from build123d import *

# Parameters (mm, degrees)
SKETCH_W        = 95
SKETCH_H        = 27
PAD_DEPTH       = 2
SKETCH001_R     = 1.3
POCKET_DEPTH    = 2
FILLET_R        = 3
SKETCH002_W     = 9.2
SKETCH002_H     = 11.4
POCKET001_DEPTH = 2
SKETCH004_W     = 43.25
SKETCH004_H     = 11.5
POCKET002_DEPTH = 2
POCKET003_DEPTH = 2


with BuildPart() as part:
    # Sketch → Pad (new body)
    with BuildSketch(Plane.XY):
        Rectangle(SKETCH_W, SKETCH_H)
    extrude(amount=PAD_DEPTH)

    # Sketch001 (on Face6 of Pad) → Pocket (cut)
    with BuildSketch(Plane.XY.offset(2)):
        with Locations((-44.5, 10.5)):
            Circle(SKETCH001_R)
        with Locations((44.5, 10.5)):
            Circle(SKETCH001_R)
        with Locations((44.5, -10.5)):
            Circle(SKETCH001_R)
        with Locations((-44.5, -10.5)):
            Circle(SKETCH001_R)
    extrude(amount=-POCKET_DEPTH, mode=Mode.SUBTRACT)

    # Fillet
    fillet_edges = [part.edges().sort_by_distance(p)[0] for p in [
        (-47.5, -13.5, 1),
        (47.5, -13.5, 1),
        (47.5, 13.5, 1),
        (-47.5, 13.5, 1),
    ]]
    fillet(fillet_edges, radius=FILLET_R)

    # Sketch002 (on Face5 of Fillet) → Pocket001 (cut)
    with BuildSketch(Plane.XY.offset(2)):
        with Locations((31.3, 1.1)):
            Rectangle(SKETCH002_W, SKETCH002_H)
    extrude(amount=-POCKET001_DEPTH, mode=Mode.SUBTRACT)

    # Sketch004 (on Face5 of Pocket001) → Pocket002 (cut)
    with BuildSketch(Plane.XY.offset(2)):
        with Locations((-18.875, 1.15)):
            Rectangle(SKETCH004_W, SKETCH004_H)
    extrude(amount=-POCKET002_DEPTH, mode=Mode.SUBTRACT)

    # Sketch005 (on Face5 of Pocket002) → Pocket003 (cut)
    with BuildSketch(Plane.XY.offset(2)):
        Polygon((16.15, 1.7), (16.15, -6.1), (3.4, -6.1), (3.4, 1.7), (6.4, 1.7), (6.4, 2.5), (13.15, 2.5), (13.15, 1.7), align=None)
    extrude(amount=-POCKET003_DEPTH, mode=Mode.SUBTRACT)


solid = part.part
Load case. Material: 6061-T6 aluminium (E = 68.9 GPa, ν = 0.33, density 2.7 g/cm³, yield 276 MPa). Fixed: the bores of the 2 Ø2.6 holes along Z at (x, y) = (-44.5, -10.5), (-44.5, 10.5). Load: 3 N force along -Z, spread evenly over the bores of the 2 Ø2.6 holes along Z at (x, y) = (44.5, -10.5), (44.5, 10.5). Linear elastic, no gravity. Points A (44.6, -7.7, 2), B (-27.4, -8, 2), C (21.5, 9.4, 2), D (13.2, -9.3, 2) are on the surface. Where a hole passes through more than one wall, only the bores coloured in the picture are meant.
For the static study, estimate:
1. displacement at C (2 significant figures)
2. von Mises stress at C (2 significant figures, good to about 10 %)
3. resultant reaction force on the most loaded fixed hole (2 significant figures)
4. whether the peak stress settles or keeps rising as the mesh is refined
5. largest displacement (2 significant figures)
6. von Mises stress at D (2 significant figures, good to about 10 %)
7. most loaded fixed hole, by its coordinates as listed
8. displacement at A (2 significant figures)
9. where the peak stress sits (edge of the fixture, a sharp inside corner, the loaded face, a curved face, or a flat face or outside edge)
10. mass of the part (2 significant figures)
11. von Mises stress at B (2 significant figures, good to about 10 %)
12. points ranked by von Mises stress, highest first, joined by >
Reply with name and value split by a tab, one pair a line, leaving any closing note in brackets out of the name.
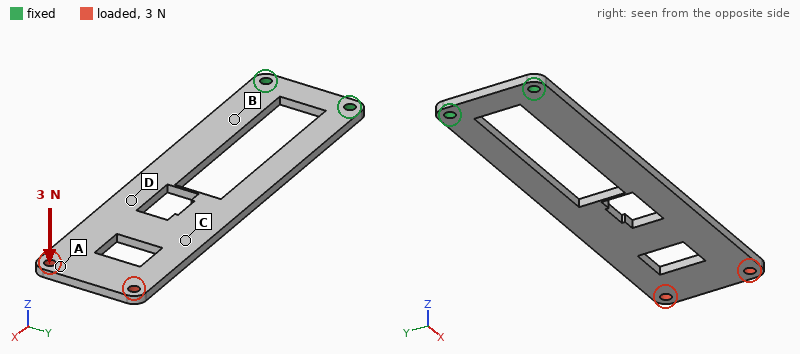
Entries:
displacement at C	0.60 mm
von Mises stress at C	4.6 MPa
resultant reaction force on the most loaded fixed hole	2.1 N
whether the peak stress settles or keeps rising as the mesh is refined	keeps rising
largest displacement	1.0 mm
von Mises stress at D	9.0 MPa
most loaded fixed hole, by its coordinates as listed	(-44.5, -10.5)
displacement at A	0.95 mm
where the peak stress sits	edge of the fixture
mass of the part	9.9 g
von Mises stress at B	21 MPa
points ranked by von Mises stress, highest first, joined by >	B > D > C > A
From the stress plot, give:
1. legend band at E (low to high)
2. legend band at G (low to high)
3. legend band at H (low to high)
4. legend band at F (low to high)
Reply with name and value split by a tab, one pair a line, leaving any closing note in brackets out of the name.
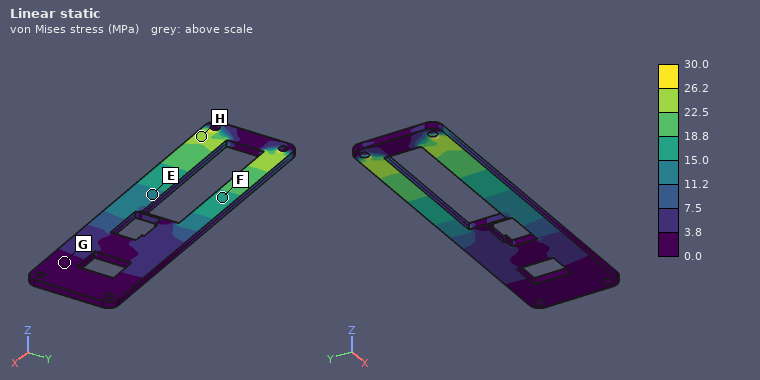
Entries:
legend band at E	11.2 to 15.0 MPa
legend band at G	0.0 to 3.8 MPa
legend band at H	22.5 to 26.2 MPa
legend band at F	15.0 to 18.8 MPa
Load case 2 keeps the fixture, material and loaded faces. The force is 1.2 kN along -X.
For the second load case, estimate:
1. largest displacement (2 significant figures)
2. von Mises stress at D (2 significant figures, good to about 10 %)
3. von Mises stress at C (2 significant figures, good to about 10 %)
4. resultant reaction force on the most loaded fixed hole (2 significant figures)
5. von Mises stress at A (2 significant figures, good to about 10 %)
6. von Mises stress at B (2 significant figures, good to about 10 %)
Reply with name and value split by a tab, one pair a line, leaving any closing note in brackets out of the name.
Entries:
largest displacement	60 µm
von Mises stress at D	43 MPa
von Mises stress at C	34 MPa
resultant reaction force on the most loaded fixed hole	610 N
von Mises stress at A	29 MPa
von Mises stress at B	33 MPa
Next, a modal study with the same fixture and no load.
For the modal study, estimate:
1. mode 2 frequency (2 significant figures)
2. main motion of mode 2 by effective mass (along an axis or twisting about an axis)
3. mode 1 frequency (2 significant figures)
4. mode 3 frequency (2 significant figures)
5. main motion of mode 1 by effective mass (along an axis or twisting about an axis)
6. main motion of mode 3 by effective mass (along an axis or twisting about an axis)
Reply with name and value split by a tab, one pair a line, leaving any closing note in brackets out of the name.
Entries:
mode 2 frequency	1000 Hz
main motion of mode 2 by effective mass	twisting about X
mode 1 frequency	160 Hz
mode 3 frequency	1100 Hz
main motion of mode 1 by effective mass	along Z
main motion of mode 3 by effective mass	along Z
